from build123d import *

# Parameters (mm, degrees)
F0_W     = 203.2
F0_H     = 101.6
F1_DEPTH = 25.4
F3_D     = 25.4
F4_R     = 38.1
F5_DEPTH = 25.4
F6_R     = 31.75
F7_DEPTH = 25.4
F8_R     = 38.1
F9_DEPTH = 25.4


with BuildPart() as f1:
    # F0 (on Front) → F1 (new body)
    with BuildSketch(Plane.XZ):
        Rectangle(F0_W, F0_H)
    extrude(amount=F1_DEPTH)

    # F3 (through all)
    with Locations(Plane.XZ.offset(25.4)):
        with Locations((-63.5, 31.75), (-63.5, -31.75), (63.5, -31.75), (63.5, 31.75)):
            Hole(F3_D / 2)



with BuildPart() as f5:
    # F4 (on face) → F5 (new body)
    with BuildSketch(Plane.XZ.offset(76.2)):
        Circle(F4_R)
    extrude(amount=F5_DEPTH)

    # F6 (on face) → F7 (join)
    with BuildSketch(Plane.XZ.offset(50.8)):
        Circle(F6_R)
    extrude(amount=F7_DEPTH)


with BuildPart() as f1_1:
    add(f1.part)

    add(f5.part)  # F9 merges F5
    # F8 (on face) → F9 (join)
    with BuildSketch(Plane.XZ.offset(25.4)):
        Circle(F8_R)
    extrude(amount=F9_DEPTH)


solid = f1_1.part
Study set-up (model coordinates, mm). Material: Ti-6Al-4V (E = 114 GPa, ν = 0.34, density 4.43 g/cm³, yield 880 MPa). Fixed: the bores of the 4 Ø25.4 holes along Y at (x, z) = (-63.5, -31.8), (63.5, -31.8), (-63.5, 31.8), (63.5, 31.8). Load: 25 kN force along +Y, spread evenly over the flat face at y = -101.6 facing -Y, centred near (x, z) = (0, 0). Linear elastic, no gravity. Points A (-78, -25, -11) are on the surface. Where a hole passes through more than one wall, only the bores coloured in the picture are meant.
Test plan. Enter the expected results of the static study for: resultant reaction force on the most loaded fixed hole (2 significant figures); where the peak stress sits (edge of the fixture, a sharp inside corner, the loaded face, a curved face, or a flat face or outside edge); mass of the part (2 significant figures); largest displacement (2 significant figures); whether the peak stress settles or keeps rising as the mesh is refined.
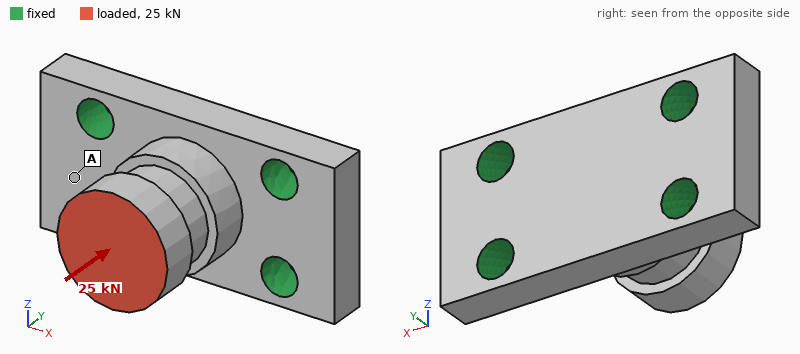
6.7 kN
edge of the fixture
3.5 kg
12 µm
keeps rising
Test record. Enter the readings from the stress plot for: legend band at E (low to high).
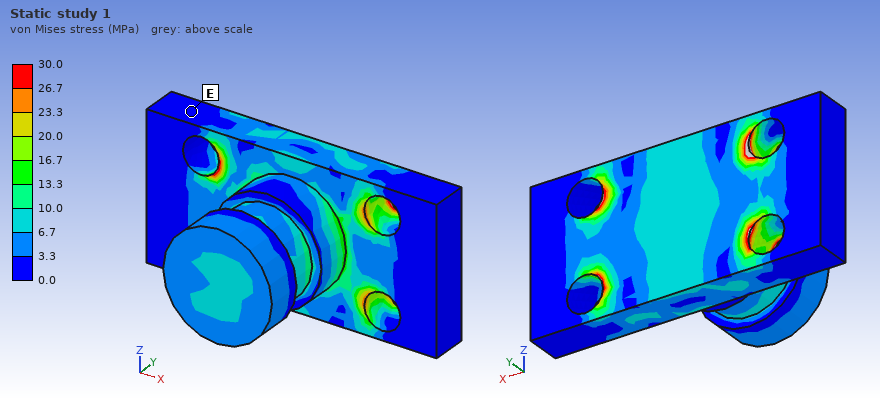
0.0 to 3.3 MPa
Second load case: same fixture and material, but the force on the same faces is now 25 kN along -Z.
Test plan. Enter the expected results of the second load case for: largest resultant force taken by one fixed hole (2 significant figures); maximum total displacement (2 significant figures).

18 kN
0.12 mm
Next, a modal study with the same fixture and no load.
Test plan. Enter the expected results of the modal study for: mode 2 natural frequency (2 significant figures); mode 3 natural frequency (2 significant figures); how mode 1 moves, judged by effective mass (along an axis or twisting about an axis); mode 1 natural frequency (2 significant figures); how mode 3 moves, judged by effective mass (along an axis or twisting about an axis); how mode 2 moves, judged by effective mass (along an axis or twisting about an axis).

4300 Hz
5900 Hz
along Z
3200 Hz
along Y
along X
